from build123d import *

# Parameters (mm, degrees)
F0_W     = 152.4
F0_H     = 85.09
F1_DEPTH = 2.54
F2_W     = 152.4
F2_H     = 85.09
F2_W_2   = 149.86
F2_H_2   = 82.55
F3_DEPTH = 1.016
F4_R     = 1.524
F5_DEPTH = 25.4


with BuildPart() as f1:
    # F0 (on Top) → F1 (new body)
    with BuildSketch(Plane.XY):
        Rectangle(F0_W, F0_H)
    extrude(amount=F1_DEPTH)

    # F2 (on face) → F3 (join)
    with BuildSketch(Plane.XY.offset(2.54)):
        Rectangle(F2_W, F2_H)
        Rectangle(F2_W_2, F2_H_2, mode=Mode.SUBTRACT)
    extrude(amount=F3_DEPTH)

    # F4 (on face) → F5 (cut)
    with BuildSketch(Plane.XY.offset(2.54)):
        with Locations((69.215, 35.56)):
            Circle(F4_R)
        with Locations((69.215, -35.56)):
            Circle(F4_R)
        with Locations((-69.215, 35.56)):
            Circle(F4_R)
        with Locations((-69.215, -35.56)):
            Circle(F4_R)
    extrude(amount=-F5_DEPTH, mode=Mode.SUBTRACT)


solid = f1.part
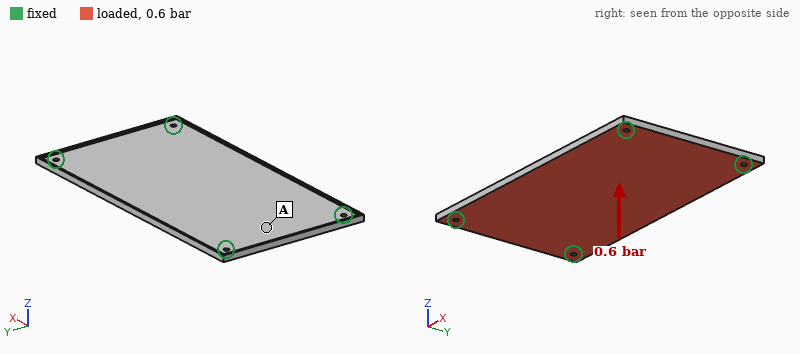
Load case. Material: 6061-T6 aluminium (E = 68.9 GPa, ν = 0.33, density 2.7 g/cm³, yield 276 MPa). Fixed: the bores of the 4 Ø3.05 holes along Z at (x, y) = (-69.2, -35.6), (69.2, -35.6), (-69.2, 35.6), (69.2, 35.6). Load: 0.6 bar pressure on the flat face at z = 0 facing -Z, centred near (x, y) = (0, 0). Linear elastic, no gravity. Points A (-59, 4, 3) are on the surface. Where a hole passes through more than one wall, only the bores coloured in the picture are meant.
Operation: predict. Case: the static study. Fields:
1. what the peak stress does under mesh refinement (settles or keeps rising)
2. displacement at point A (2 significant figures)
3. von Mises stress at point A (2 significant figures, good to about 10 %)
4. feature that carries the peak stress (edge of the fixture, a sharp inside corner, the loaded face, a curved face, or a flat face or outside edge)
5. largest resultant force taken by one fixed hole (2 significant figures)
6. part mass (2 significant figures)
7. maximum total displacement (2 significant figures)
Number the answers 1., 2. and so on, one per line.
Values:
1. keeps rising
2. 0.19 mm
3. 24 MPa
4. edge of the fixture
5. 190 N
6. 90 g
7. 0.80 mm
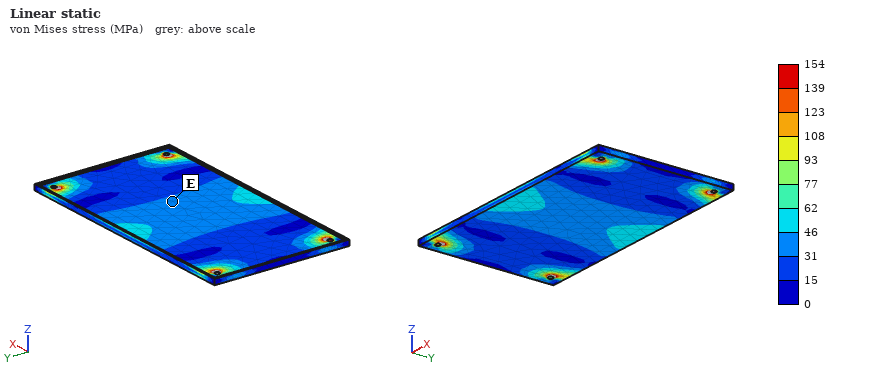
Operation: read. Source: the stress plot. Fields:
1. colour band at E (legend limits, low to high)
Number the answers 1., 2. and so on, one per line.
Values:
1. 31 to 46 MPa
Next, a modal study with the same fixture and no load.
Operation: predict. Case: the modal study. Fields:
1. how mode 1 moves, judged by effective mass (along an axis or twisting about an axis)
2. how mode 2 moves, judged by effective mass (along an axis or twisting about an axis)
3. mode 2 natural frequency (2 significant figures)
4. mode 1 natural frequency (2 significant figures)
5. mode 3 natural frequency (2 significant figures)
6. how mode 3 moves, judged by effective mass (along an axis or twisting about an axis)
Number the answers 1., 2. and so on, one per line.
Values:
1. along Z
2. twisting about X
3. 1000 Hz
4. 600 Hz
5. 1600 Hz
6. twisting about Y
